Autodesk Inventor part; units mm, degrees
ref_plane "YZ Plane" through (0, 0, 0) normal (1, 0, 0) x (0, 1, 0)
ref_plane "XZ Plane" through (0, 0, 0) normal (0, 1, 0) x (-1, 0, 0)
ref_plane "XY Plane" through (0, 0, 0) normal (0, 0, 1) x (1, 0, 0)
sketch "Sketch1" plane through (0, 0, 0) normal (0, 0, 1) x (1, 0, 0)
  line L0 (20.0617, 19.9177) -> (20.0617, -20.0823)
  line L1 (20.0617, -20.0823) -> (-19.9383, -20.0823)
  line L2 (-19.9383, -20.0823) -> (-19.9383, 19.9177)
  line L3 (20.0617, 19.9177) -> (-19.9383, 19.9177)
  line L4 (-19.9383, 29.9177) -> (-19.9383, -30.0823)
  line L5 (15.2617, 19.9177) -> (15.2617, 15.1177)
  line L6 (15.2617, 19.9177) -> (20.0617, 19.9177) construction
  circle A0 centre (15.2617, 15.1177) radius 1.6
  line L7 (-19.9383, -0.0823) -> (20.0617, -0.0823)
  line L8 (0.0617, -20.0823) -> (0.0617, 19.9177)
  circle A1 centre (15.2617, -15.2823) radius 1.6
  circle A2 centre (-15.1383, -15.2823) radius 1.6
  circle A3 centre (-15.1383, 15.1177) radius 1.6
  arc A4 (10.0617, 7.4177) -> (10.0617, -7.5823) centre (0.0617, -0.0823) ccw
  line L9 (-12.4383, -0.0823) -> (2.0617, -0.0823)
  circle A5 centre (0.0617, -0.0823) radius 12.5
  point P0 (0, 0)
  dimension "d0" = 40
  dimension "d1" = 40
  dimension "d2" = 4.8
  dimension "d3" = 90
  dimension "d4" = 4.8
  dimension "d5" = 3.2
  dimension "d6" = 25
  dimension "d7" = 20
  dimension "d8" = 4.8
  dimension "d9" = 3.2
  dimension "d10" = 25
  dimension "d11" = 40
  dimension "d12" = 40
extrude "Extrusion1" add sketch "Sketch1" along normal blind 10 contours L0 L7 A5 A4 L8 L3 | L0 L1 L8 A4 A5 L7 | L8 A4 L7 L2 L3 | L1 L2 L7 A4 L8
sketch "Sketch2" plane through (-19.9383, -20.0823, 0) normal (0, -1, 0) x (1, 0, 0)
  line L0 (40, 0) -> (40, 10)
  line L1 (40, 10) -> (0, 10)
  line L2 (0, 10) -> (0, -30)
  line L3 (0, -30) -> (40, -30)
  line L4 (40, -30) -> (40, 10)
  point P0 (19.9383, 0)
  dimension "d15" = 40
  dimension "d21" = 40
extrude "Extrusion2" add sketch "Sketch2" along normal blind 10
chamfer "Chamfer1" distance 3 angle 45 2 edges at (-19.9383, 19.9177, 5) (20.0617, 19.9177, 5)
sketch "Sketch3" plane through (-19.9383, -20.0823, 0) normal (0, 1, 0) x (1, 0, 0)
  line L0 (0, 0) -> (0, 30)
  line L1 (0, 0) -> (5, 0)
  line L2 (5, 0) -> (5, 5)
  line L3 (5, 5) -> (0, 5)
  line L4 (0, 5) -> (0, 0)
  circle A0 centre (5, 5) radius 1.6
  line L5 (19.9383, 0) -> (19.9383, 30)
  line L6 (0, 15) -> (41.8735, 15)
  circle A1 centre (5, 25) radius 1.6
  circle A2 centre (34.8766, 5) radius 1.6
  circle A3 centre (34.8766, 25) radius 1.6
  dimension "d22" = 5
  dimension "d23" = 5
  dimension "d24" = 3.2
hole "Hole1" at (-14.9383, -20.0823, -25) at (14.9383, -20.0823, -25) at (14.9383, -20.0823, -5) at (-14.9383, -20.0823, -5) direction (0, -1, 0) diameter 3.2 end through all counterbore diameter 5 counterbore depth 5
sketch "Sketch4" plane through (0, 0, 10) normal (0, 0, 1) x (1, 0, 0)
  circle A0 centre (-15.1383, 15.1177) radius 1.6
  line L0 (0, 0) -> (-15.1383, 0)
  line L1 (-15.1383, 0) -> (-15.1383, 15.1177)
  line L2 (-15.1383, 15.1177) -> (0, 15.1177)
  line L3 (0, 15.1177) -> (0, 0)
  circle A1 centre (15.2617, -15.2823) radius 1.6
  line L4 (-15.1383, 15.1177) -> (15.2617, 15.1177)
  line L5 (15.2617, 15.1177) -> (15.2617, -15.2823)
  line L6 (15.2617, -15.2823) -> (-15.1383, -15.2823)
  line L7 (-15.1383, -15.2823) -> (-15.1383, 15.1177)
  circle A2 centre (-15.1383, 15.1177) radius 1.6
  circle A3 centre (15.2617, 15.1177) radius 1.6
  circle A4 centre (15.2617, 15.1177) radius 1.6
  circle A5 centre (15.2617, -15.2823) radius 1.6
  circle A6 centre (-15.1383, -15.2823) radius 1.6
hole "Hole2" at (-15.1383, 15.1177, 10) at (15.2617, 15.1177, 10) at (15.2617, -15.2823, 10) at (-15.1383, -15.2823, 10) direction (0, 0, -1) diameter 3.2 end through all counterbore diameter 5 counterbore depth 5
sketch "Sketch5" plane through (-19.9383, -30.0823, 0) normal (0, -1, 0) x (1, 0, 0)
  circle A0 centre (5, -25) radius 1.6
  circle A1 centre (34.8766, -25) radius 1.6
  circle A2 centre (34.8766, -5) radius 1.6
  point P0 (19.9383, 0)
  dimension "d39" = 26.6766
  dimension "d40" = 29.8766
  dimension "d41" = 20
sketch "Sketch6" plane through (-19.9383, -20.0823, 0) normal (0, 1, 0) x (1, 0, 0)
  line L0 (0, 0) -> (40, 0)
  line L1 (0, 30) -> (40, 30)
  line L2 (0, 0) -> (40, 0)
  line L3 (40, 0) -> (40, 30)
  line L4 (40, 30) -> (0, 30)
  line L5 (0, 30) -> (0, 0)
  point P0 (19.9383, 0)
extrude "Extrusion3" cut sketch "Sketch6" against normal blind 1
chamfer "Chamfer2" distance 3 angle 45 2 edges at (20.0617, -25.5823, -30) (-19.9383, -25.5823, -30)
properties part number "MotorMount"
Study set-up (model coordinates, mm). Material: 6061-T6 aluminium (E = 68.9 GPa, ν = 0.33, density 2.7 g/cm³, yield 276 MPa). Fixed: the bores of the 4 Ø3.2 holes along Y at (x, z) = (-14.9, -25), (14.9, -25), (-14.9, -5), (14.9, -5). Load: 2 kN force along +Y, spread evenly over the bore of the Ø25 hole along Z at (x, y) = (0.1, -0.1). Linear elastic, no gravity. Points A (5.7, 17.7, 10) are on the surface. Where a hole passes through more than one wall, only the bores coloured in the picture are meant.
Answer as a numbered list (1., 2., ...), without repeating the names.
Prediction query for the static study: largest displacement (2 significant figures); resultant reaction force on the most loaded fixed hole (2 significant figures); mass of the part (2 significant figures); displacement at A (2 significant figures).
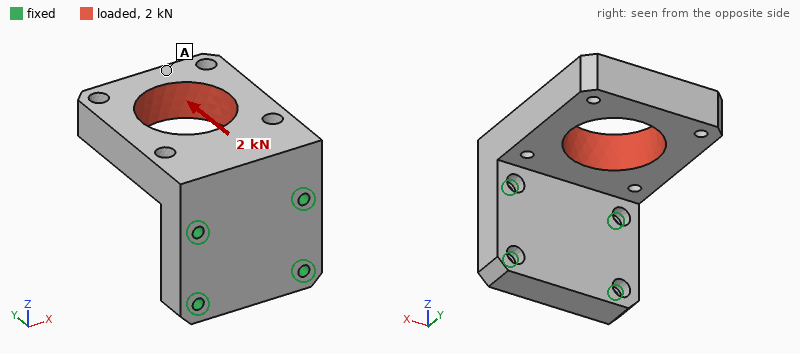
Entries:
1. 70 µm
2. 1.4 kN
3. 67 g
4. 67 µm
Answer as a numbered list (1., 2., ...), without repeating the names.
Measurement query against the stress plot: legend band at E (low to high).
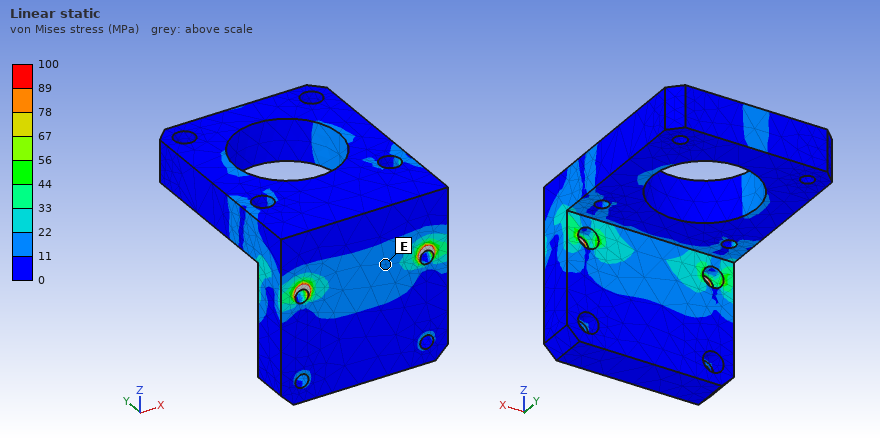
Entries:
1. 11 to 22 MPa
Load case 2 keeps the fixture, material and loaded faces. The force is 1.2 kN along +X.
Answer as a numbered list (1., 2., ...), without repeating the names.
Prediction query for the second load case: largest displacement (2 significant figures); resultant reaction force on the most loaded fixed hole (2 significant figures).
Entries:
1. 48 µm
2. 1.3 kN
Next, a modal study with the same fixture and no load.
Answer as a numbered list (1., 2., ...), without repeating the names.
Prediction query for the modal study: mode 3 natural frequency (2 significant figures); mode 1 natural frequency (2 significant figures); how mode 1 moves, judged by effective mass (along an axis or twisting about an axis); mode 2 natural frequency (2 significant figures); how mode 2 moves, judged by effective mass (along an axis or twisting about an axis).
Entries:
1. 7200 Hz
2. 2600 Hz
3. along Z
4. 5200 Hz
5. along X
